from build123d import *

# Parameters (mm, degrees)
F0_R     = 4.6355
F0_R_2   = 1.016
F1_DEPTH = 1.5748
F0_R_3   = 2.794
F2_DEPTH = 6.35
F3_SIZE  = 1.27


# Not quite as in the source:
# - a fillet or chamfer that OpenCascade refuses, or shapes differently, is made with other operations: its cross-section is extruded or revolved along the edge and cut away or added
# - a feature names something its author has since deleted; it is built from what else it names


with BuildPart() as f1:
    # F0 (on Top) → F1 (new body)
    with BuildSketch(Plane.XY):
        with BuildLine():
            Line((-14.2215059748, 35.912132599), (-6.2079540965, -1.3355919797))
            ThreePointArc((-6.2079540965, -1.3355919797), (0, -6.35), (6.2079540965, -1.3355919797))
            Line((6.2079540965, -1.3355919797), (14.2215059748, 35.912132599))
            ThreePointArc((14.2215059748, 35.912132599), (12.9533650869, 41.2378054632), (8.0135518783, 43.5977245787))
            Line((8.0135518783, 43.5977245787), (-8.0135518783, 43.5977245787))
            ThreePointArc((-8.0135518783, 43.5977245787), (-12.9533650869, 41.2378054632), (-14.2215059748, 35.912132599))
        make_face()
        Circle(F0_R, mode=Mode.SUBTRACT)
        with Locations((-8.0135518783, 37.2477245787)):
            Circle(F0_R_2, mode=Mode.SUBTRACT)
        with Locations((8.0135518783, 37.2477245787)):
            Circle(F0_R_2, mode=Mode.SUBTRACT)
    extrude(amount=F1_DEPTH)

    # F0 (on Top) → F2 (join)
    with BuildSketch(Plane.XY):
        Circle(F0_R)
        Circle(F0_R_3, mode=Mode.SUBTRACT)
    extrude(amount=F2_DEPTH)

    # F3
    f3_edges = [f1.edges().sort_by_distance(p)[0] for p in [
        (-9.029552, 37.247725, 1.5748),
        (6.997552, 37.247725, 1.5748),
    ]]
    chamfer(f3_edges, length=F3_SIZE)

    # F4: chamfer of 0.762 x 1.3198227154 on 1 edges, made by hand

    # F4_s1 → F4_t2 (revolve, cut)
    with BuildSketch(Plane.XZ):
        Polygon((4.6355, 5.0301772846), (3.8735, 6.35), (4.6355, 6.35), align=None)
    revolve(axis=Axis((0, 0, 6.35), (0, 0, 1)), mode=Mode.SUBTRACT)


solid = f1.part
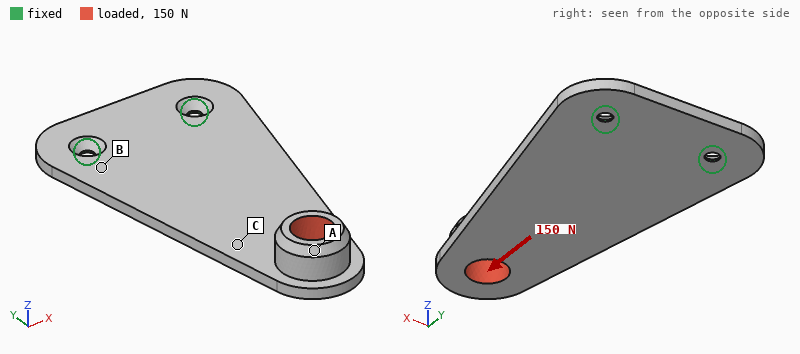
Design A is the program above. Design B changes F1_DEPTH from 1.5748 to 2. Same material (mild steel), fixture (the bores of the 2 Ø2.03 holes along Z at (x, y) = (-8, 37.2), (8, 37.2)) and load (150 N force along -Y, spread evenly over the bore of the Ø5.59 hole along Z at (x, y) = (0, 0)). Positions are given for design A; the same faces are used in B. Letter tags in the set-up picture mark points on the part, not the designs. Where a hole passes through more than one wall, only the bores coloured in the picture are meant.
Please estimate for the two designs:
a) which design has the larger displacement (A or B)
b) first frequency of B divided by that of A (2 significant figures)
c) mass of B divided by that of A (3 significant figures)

A
1.5
1.23
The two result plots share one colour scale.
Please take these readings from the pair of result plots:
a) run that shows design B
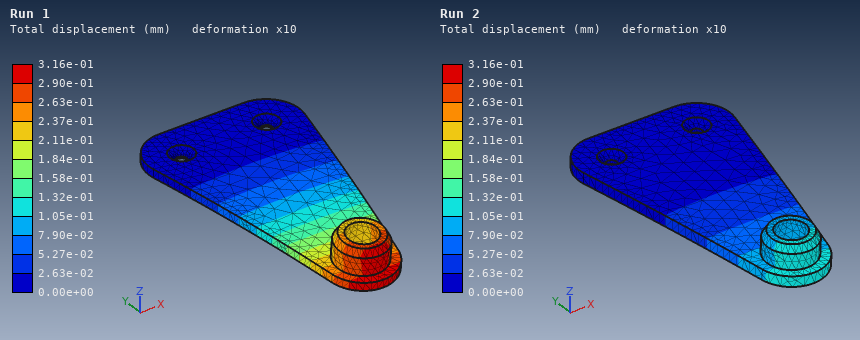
Run 2
